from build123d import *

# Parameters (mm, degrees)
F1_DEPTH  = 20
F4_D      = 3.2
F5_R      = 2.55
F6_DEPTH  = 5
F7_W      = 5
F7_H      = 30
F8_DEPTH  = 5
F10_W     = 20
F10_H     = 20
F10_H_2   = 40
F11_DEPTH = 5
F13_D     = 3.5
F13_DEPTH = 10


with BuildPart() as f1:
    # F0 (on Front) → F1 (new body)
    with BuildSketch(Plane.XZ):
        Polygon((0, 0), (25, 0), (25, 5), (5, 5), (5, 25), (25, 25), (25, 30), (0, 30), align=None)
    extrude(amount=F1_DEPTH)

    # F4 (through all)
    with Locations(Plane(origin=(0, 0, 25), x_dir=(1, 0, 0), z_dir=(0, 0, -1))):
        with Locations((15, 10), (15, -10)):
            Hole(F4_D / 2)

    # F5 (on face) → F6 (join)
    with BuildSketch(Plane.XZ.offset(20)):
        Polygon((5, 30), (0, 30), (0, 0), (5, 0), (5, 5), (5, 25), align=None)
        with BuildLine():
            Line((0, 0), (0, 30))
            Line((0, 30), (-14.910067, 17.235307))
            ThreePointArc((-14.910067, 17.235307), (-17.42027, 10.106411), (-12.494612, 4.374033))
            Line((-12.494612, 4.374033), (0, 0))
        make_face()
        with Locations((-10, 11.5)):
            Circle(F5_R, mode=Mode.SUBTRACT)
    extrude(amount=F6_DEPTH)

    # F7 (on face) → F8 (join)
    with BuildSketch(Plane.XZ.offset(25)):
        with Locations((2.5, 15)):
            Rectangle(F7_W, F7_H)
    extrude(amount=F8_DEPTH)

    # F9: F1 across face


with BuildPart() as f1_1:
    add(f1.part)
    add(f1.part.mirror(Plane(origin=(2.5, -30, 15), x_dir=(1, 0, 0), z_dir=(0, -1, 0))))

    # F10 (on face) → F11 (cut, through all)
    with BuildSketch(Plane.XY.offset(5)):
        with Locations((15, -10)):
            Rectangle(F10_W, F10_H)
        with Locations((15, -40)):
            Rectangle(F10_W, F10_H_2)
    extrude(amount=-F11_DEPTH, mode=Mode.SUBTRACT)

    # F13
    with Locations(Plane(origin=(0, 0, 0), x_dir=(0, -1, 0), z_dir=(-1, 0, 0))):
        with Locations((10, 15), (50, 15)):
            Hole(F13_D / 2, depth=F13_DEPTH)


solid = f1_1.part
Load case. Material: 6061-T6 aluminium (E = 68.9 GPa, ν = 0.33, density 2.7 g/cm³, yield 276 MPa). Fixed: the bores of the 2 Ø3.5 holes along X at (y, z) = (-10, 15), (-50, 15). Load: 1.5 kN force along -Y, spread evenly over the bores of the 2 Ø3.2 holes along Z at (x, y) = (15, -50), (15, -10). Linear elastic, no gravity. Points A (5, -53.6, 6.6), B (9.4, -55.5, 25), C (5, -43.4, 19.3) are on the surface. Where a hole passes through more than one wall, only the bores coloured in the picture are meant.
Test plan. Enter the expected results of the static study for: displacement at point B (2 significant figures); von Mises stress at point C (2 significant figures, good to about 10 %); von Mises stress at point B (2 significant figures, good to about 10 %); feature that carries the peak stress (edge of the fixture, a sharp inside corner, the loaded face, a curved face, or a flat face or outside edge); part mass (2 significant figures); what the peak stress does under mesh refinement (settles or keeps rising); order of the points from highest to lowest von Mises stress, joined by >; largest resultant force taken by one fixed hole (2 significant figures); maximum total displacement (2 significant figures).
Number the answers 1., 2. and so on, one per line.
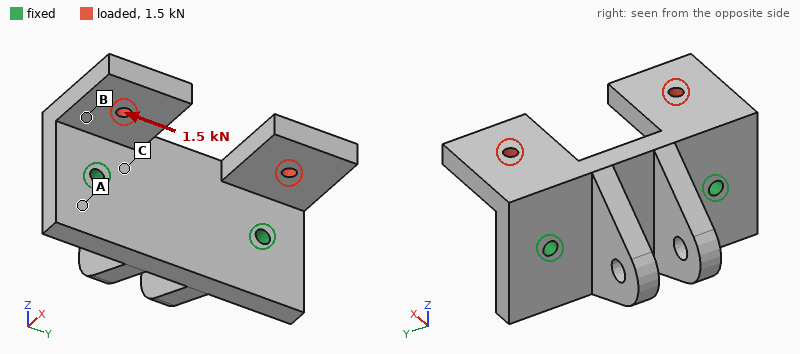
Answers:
1. 32 µm
2. 32 MPa
3. 22 MPa
4. edge of the fixture
5. 43 g
6. keeps rising
7. C > B > A
8. 930 N
9. 74 µm
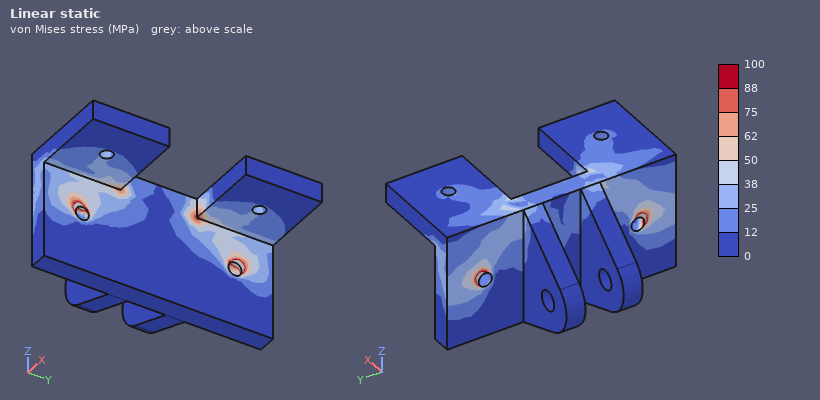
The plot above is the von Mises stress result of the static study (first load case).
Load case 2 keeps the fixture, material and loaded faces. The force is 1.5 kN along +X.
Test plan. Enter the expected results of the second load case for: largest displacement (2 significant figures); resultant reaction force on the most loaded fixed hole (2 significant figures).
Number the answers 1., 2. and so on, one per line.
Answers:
1. 96 µm
2. 750 N
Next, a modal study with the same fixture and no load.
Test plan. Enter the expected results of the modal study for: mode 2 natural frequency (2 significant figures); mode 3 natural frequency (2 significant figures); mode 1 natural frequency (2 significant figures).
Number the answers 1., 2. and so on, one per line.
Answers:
1. 5200 Hz
2. 6200 Hz
3. 4400 Hz
